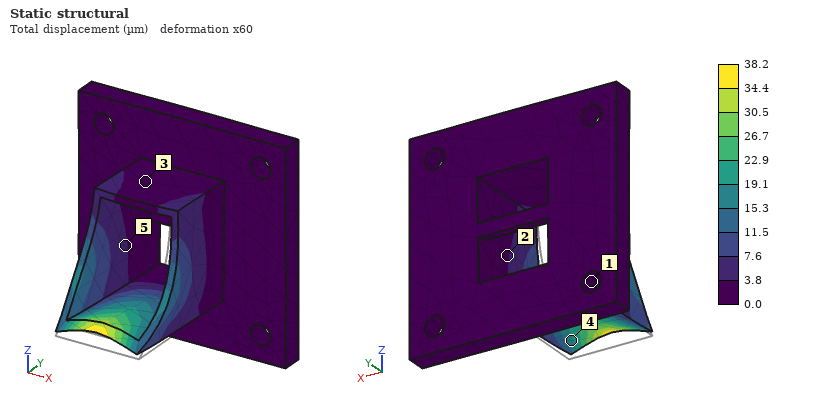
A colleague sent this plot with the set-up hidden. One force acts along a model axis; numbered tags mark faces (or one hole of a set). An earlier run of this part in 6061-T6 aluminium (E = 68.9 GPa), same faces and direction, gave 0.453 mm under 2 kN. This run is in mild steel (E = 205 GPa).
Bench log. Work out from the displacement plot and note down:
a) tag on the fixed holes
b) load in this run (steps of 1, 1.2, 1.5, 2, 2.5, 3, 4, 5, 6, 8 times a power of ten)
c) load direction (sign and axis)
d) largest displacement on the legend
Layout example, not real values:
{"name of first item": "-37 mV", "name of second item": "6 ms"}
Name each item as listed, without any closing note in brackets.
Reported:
{"tag on the fixed holes": "1", "load in this run": "500 N", "load direction": "+Z", "largest displacement on the legend": "38.2 µm"}
